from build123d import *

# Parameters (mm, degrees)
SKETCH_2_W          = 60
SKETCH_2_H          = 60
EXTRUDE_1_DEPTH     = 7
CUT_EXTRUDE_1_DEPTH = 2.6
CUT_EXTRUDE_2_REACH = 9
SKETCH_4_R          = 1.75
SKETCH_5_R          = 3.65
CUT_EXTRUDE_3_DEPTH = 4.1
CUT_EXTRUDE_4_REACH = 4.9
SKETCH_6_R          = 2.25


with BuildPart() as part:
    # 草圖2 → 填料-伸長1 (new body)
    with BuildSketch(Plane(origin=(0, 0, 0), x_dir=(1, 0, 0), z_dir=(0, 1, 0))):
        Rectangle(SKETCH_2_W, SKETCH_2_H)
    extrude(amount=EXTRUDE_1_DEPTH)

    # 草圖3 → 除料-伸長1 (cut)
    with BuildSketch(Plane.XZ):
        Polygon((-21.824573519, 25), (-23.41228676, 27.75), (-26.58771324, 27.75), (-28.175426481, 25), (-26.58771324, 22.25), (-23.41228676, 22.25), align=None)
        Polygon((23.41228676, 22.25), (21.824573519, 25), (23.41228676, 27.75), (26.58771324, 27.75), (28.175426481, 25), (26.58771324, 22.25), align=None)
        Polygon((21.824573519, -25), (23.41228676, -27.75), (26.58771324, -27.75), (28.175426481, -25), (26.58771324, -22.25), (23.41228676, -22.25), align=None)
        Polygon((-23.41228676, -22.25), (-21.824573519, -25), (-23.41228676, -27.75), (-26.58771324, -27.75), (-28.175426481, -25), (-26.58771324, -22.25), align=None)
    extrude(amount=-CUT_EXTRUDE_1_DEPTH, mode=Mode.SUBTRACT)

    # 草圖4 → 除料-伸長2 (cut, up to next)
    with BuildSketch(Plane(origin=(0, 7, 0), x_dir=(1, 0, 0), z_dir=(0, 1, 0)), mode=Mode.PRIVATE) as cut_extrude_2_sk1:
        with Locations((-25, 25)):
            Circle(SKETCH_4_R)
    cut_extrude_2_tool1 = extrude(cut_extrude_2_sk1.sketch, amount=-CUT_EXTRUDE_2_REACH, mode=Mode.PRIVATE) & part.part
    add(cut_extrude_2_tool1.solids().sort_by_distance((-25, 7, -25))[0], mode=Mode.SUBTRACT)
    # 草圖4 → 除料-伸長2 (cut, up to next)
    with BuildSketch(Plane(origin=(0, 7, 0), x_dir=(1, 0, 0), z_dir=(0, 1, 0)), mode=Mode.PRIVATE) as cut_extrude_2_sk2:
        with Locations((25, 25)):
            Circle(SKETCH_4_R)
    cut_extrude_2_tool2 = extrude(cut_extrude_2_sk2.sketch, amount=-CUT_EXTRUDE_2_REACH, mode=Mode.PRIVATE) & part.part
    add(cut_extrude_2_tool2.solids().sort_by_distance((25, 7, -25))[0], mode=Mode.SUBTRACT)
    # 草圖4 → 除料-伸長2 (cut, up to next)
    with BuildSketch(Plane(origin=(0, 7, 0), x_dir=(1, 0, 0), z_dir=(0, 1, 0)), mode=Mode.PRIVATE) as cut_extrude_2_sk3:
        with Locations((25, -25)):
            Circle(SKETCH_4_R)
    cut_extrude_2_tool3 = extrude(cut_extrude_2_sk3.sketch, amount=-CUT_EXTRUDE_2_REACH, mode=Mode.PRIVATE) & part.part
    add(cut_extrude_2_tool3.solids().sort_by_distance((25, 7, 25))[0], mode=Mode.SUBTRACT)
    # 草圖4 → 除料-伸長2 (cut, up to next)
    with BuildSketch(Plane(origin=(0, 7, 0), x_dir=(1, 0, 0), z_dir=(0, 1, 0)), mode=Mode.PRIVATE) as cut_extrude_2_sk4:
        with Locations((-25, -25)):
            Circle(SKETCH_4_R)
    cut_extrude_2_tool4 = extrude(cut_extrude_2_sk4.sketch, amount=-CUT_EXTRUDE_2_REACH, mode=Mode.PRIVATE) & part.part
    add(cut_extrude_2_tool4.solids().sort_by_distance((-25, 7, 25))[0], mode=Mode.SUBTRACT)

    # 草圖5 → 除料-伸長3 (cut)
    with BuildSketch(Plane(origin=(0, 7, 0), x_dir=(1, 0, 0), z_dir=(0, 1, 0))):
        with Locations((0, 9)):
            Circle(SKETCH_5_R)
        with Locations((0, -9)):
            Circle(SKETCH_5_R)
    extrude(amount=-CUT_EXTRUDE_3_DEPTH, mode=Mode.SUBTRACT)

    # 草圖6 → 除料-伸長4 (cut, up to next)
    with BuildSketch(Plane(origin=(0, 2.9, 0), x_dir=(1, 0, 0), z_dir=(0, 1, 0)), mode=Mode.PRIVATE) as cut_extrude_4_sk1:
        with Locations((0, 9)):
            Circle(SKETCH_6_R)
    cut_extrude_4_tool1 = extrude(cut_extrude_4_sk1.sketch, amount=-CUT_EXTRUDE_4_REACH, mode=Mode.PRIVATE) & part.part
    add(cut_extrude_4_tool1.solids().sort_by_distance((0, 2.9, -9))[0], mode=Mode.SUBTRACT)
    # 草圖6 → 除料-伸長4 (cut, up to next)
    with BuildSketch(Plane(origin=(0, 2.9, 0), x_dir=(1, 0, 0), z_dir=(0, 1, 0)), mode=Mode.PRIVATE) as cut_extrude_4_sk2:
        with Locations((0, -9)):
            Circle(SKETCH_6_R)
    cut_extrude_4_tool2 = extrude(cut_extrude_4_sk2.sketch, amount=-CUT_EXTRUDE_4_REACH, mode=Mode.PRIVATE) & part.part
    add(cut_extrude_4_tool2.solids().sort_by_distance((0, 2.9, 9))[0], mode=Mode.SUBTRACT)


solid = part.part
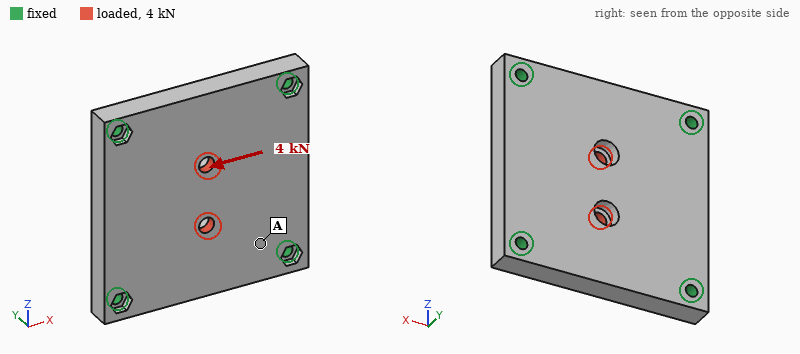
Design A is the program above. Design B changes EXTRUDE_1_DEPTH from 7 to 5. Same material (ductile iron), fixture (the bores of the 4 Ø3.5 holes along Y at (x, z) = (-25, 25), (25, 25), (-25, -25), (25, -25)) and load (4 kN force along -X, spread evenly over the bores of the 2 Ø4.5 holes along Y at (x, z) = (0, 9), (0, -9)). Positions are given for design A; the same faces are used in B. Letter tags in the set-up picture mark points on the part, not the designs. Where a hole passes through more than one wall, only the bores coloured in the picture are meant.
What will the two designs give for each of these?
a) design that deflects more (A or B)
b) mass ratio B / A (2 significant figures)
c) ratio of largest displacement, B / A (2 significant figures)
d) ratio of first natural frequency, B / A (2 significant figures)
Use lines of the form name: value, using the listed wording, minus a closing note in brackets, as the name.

design that deflects more: B
mass ratio B / A: 0.71
ratio of largest displacement, B / A: 1.3
ratio of first natural frequency, B / A: 0.74
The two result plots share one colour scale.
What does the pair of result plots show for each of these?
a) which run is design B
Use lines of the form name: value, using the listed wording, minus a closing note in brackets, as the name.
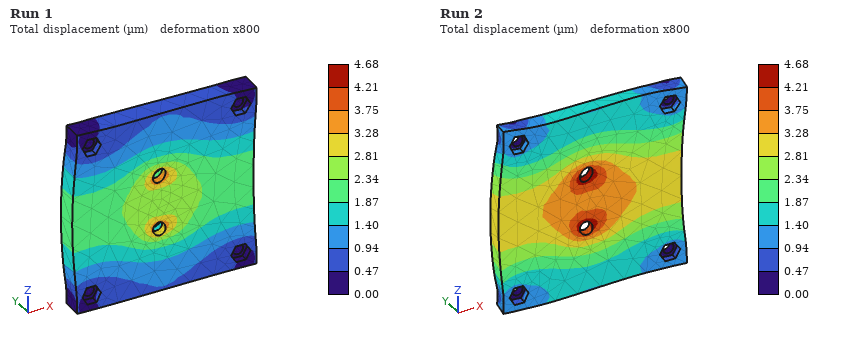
which run is design B: Run 2
